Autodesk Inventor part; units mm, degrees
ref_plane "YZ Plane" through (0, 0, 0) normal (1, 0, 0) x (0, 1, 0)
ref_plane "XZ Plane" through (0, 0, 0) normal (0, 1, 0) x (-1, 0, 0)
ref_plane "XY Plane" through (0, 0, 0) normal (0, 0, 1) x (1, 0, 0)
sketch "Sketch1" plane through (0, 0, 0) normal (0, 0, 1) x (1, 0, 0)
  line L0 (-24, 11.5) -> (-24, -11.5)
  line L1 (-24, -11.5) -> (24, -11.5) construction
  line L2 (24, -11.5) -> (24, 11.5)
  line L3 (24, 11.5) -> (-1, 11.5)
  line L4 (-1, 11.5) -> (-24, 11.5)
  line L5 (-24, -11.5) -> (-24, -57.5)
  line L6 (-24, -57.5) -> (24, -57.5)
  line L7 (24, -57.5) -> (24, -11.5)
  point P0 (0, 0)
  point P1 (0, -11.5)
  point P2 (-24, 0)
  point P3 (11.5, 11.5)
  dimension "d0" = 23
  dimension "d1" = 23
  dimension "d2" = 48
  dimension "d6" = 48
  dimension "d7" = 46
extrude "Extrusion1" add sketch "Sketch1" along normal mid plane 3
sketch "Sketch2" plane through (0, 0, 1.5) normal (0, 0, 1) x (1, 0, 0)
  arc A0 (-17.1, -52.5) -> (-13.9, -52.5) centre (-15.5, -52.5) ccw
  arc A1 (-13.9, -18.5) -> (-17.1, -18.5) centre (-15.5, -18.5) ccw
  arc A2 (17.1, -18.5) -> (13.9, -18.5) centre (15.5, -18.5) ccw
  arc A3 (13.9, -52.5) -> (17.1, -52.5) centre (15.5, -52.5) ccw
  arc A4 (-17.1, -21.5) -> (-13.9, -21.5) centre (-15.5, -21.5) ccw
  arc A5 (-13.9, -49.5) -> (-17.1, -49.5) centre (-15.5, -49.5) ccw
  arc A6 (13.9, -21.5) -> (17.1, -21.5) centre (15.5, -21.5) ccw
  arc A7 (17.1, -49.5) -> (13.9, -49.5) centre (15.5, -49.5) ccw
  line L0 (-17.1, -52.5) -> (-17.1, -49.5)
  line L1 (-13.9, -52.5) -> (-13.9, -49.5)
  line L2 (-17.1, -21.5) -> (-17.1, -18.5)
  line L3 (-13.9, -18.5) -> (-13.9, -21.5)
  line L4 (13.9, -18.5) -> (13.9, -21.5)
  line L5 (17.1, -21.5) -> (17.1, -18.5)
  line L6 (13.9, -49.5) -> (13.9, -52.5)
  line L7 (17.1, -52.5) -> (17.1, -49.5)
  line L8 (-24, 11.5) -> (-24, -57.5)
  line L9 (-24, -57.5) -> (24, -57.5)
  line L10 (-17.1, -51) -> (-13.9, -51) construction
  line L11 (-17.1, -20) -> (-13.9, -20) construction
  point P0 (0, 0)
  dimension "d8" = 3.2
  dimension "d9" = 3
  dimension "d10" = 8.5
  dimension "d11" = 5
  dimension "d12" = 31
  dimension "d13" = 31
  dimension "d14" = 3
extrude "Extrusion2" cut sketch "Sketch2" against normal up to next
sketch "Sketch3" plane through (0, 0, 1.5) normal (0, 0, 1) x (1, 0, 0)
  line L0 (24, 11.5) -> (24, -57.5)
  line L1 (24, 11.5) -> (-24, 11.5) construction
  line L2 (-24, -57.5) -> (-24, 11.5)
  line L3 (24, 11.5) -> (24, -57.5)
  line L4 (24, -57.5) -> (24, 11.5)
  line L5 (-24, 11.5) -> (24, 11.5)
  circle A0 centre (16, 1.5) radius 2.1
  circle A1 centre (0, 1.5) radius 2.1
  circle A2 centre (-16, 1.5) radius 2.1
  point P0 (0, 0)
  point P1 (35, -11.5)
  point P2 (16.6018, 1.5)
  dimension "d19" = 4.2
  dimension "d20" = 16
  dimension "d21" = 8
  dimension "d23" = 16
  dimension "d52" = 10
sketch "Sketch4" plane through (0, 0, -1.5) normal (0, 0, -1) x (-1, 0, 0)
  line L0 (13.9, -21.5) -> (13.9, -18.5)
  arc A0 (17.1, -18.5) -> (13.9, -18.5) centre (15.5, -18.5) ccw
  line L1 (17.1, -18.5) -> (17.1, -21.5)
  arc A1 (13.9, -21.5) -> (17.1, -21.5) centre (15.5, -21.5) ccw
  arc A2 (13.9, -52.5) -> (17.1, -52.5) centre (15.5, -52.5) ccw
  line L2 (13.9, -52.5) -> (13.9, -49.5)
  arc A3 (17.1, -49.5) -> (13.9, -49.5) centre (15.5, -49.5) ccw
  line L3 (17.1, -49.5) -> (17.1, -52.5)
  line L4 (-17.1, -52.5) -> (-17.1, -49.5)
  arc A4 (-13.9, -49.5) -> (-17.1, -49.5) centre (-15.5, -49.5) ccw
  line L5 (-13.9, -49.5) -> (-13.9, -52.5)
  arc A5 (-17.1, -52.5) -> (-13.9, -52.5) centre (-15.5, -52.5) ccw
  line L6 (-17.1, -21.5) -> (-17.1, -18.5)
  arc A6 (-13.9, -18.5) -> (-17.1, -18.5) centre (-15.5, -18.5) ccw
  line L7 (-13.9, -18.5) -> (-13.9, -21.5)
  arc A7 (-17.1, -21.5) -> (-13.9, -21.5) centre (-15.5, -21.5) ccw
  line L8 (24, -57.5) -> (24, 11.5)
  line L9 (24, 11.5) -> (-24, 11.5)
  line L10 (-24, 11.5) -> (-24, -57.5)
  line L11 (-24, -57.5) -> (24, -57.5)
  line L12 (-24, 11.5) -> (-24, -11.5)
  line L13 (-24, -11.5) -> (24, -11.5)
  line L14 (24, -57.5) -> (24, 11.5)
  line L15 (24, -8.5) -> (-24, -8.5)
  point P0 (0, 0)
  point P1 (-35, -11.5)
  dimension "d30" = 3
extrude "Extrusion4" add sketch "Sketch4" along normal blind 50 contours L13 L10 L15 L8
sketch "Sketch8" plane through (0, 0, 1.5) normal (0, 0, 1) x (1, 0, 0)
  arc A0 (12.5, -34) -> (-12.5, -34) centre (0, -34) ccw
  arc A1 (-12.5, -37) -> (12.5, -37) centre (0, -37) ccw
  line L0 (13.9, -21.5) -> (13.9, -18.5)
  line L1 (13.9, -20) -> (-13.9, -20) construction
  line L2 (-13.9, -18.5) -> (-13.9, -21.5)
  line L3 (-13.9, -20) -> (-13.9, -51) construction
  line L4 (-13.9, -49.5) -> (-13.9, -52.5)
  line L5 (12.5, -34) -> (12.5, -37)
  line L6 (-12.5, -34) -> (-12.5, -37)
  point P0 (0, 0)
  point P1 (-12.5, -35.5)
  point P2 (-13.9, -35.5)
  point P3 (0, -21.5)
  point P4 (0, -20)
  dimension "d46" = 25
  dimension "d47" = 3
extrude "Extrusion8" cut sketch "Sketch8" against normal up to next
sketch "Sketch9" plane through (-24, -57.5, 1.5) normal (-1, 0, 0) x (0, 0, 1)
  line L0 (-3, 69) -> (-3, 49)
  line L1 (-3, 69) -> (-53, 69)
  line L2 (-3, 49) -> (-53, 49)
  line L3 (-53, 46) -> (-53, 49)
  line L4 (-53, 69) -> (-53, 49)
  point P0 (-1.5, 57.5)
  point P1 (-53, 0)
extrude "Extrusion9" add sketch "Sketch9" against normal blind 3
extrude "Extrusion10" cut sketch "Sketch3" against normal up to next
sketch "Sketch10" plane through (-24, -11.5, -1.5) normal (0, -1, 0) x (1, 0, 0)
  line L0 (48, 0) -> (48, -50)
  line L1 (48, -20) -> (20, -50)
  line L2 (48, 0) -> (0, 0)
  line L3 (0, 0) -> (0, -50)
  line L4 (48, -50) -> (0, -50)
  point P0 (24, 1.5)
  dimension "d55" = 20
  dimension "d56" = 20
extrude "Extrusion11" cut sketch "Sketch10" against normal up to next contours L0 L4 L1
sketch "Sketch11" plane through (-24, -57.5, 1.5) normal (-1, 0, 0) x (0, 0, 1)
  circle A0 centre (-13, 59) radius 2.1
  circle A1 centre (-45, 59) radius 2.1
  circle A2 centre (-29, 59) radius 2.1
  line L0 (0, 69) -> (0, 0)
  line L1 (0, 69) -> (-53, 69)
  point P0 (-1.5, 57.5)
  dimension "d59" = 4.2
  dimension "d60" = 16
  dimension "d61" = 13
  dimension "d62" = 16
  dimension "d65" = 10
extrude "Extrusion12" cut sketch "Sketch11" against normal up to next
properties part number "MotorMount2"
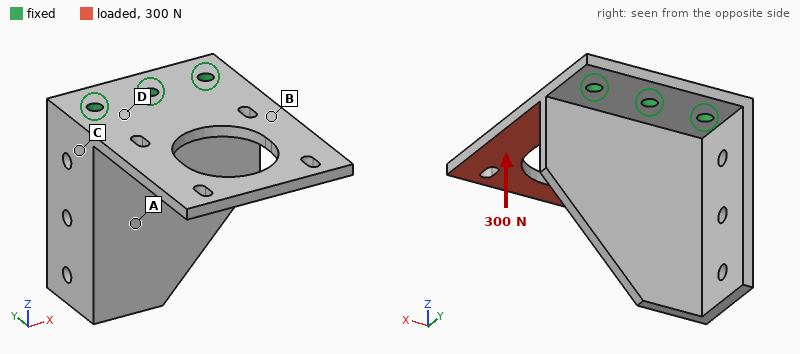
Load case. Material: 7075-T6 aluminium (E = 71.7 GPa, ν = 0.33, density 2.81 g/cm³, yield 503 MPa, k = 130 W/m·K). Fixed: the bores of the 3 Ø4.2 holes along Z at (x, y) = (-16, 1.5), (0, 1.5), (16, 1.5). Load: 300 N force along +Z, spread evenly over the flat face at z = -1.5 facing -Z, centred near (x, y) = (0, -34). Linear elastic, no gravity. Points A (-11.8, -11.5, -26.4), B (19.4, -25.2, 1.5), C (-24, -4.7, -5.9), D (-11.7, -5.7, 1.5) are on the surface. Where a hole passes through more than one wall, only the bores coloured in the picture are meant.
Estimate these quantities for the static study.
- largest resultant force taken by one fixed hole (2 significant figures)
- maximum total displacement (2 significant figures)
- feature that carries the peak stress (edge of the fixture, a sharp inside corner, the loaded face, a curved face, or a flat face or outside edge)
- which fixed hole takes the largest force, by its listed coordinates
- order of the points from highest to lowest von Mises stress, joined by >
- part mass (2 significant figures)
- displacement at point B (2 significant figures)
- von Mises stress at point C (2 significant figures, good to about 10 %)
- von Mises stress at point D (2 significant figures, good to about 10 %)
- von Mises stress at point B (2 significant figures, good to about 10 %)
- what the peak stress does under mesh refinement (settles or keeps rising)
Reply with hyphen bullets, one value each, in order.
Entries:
- 150 N
- 1.2 mm
- edge of the fixture
- (0, 1.5)
- B > D > C > A
- 47 g
- 0.28 mm
- 23 MPa
- 59 MPa
- 75 MPa
- keeps rising
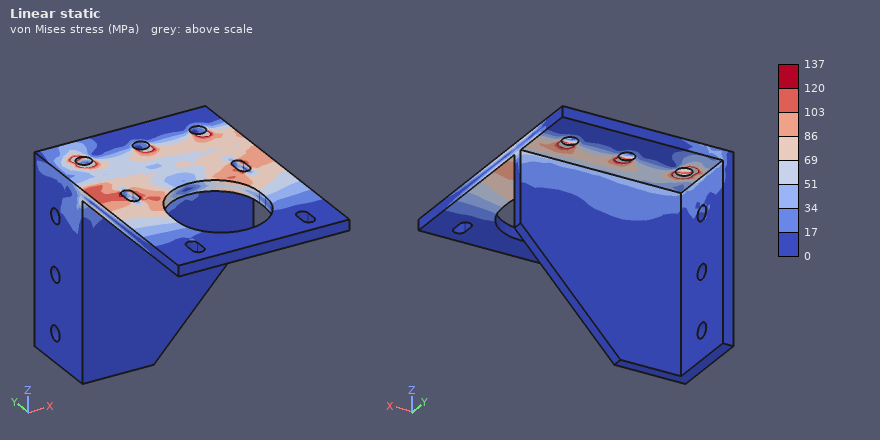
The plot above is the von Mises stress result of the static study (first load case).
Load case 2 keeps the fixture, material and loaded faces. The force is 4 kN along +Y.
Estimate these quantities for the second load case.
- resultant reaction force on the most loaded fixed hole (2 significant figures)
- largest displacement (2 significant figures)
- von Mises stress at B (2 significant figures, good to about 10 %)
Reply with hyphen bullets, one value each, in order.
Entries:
- 1.6 kN
- 1.1 mm
- 50 MPa
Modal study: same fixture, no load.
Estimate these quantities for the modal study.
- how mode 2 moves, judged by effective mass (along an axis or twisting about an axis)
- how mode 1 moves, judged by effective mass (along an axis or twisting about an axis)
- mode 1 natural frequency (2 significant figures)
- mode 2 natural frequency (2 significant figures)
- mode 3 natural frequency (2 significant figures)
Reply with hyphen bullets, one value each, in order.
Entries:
- along Y
- along Z
- 810 Hz
- 1500 Hz
- 1900 Hz
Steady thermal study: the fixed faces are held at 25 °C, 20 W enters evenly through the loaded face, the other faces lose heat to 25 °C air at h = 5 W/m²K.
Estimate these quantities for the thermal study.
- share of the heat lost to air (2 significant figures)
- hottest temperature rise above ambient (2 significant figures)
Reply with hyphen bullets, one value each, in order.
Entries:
- 3.8 %
- 53 K
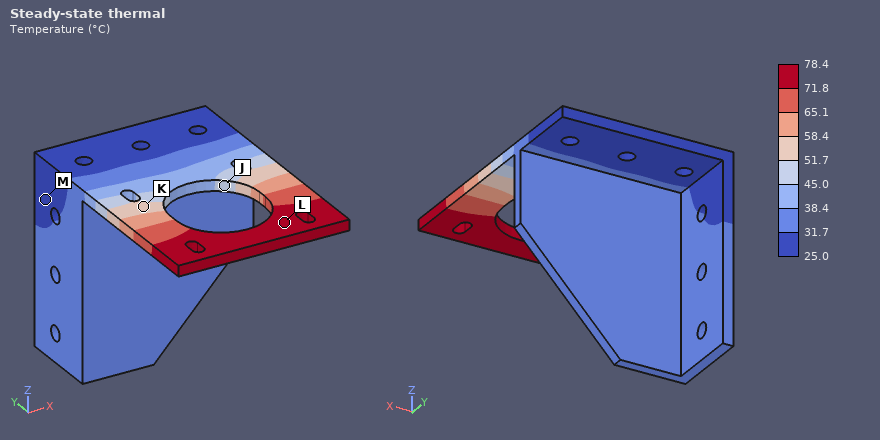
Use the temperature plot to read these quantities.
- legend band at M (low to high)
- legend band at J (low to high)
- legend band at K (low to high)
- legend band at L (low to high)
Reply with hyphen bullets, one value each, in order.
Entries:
- 25.0 to 31.7 °C
- 45.0 to 51.7 °C
- 51.7 to 58.4 °C
- 71.8 to 78.4 °C
